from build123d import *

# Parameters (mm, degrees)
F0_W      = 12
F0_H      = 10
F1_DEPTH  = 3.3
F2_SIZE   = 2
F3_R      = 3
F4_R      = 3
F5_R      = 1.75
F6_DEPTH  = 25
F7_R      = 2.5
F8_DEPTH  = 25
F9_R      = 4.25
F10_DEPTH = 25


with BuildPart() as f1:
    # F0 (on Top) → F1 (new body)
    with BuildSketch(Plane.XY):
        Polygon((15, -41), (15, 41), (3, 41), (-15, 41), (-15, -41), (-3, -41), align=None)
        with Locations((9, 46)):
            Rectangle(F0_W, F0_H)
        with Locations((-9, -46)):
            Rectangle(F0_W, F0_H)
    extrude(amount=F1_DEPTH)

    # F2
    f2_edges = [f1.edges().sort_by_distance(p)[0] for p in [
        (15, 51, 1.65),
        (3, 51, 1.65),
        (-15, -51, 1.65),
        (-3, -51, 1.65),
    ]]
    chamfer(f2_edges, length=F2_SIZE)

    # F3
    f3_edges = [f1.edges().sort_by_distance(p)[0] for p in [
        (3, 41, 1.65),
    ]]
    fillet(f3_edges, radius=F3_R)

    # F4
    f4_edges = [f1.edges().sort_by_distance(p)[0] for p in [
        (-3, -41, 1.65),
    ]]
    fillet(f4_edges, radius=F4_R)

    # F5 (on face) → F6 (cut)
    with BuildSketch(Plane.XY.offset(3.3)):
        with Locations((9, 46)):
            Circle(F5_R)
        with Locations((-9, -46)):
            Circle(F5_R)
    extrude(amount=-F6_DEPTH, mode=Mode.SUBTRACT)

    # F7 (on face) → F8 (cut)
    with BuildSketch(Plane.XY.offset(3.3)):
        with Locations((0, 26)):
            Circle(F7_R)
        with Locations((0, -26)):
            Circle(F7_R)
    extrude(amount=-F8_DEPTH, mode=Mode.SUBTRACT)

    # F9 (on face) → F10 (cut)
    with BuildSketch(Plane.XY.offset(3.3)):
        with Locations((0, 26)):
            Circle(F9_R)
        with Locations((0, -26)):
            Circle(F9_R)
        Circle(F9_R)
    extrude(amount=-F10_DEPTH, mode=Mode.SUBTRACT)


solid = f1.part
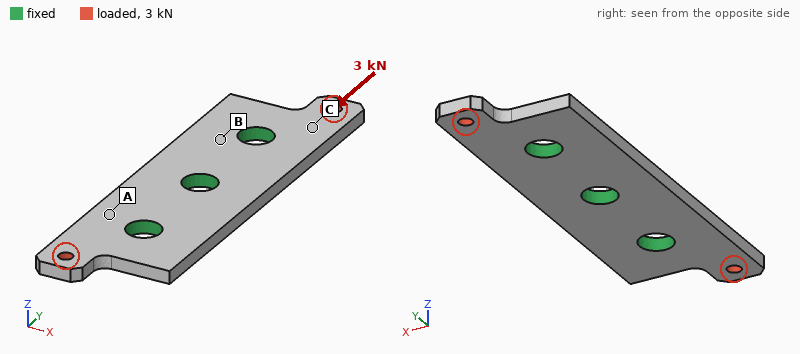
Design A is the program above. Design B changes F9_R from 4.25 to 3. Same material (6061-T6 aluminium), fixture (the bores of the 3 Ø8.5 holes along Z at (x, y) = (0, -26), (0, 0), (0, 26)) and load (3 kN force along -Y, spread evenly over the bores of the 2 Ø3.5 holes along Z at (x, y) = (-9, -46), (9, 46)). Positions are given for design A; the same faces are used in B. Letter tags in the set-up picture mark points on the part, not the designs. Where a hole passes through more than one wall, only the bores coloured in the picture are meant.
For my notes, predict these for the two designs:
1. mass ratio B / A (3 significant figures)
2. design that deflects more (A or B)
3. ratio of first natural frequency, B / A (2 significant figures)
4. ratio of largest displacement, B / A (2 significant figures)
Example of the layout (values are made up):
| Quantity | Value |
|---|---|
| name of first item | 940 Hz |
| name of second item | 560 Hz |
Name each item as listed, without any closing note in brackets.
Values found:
| Quantity | Value |
|---|---|
| mass ratio B / A | 1.03 |
| design that deflects more | B |
| ratio of first natural frequency, B / A | 0.90 |
| ratio of largest displacement, B / A | 1.1 |
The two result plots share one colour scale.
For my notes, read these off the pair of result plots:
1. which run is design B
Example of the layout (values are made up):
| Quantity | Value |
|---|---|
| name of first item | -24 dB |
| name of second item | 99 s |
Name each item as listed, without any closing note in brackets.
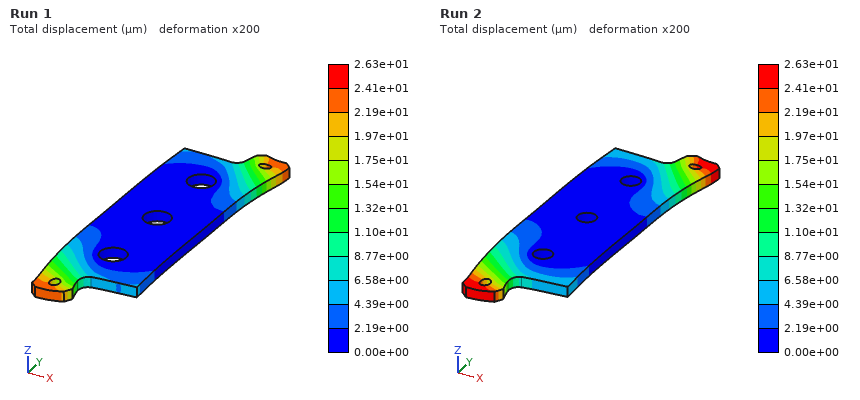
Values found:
| Quantity | Value |
|---|---|
| which run is design B | Run 2 |
